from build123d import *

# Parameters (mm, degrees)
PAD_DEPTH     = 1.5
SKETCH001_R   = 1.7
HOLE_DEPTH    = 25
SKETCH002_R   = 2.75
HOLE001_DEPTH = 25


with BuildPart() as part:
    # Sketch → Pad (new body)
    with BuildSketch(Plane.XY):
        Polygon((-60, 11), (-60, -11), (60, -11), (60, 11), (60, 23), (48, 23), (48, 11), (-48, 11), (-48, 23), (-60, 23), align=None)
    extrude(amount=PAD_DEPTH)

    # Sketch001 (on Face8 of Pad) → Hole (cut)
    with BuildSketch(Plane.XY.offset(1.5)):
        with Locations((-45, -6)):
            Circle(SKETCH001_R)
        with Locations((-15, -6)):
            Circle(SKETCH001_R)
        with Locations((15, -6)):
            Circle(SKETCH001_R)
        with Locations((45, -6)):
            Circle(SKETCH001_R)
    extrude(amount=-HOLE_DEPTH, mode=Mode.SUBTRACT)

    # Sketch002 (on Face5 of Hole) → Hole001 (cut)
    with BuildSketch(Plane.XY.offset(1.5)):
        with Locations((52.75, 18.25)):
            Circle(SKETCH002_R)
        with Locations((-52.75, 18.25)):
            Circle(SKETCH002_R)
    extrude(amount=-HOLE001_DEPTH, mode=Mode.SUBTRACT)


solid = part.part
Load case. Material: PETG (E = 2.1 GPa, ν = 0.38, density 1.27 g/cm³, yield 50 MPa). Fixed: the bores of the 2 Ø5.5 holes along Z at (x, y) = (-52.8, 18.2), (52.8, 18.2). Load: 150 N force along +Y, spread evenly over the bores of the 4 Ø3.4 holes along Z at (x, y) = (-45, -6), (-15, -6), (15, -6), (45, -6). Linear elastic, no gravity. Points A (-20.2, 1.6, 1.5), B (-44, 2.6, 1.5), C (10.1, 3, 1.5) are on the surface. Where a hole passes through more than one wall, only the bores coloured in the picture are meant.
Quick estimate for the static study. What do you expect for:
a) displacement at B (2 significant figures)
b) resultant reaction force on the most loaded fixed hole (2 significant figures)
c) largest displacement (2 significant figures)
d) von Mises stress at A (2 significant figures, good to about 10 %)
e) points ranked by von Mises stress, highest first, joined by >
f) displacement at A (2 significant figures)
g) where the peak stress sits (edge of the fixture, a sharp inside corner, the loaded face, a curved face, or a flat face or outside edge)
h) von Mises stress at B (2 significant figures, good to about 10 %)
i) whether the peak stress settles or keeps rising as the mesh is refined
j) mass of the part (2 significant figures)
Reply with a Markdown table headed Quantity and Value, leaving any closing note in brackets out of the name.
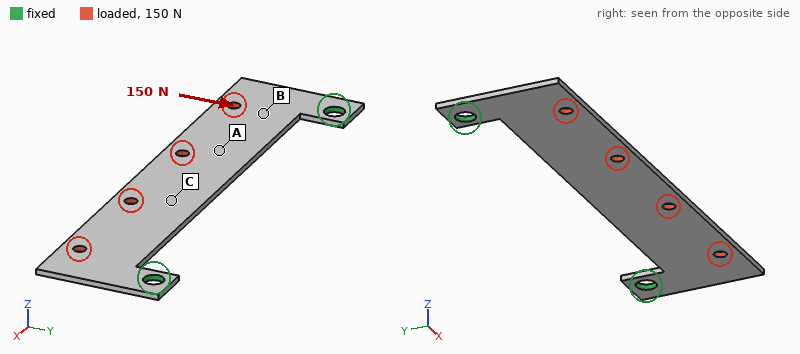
| Quantity | Value |
|---|---|
| displacement at B | 0.097 mm |
| resultant reaction force on the most loaded fixed hole | 93 N |
| largest displacement | 0.39 mm |
| von Mises stress at A | 3.0 MPa |
| points ranked by von Mises stress, highest first, joined by > | B > A > C |
| displacement at A | 0.32 mm |
| where the peak stress sits | a sharp inside corner |
| von Mises stress at B | 5.1 MPa |
| whether the peak stress settles or keeps rising as the mesh is refined | keeps rising |
| mass of the part | 5.4 g |
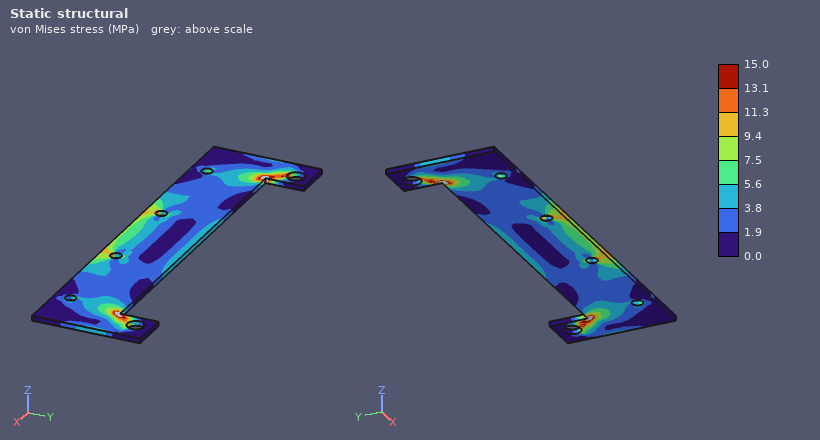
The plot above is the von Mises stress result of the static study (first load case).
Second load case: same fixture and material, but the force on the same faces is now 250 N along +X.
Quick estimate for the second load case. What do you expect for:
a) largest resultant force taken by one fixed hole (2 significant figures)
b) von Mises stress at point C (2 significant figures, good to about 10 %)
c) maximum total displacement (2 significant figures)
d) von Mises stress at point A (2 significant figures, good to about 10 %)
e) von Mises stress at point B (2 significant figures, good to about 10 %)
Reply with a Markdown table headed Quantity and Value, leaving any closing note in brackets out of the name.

| Quantity | Value |
|---|---|
| largest resultant force taken by one fixed hole | 130 N |
| von Mises stress at point C | 3.1 MPa |
| maximum total displacement | 0.35 mm |
| von Mises stress at point A | 3.7 MPa |
| von Mises stress at point B | 4.4 MPa |
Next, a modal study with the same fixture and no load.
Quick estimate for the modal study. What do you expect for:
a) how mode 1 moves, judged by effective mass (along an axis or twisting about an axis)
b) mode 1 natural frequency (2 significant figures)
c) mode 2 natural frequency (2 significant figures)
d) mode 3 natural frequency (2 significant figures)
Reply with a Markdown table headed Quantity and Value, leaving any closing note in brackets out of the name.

| Quantity | Value |
|---|---|
| how mode 1 moves, judged by effective mass | along Z |
| mode 1 natural frequency | 120 Hz |
| mode 2 natural frequency | 310 Hz |
| mode 3 natural frequency | 310 Hz |
